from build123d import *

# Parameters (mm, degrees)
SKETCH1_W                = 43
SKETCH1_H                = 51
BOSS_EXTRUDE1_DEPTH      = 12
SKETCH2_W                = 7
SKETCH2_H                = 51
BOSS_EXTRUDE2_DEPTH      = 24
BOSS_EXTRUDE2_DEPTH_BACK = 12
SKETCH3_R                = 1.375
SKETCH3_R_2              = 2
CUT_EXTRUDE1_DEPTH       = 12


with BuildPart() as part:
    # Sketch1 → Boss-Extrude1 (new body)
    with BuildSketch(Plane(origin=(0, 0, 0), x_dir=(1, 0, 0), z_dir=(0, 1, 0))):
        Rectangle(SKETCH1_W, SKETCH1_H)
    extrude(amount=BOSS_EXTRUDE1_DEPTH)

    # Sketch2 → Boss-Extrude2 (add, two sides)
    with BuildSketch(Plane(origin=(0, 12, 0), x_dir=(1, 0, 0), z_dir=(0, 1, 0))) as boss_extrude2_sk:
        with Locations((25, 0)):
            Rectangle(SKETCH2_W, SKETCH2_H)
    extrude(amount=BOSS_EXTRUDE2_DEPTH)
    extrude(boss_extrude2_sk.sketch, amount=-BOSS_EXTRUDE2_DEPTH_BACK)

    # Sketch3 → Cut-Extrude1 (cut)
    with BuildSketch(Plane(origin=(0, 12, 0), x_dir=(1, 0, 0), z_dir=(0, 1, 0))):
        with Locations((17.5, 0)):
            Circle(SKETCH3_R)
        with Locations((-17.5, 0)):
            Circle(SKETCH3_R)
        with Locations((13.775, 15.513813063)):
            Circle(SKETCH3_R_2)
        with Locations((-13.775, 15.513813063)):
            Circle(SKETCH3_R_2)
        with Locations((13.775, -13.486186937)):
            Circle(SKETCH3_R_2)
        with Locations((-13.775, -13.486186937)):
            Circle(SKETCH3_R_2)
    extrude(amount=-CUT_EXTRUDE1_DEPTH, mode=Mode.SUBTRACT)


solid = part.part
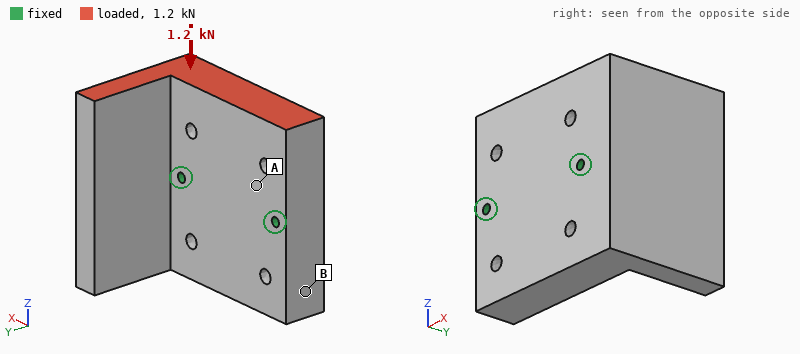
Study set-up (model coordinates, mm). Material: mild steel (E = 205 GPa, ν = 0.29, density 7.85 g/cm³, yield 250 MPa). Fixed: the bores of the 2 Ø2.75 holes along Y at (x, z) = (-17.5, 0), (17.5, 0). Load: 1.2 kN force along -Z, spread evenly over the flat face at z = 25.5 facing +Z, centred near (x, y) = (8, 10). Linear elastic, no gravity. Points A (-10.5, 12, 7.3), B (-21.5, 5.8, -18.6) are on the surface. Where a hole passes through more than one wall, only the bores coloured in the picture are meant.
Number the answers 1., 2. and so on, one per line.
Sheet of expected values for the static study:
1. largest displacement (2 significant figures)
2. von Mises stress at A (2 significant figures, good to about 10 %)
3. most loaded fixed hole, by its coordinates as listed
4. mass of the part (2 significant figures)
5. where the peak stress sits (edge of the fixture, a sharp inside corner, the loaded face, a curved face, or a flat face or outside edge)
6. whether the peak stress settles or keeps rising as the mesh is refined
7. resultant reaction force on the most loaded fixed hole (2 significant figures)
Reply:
1. 2.6 µm
2. 3.0 MPa
3. (17.5, 0)
4. 300 g
5. edge of the fixture
6. keeps rising
7. 870 N
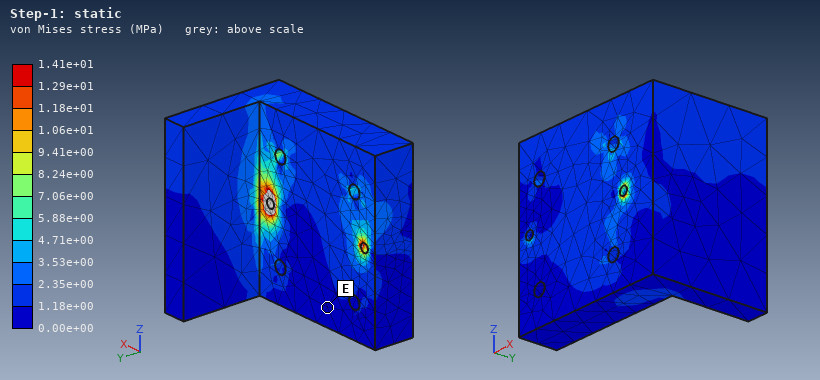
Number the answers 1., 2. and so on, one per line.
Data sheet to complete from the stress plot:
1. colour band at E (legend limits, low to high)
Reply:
1. 0.00e+00 to 1.18e+00 MPa
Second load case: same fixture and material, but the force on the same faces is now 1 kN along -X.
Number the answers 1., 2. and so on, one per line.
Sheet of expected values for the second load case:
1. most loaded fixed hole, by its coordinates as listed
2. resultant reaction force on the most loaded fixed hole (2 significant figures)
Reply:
1. (17.5, 0)
2. 920 N
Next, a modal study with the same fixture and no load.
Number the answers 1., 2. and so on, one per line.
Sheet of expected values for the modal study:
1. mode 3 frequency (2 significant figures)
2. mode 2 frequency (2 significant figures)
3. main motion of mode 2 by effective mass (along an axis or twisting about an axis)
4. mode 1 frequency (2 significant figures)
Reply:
1. 9600 Hz
2. 6100 Hz
3. along X
4. 5800 Hz
